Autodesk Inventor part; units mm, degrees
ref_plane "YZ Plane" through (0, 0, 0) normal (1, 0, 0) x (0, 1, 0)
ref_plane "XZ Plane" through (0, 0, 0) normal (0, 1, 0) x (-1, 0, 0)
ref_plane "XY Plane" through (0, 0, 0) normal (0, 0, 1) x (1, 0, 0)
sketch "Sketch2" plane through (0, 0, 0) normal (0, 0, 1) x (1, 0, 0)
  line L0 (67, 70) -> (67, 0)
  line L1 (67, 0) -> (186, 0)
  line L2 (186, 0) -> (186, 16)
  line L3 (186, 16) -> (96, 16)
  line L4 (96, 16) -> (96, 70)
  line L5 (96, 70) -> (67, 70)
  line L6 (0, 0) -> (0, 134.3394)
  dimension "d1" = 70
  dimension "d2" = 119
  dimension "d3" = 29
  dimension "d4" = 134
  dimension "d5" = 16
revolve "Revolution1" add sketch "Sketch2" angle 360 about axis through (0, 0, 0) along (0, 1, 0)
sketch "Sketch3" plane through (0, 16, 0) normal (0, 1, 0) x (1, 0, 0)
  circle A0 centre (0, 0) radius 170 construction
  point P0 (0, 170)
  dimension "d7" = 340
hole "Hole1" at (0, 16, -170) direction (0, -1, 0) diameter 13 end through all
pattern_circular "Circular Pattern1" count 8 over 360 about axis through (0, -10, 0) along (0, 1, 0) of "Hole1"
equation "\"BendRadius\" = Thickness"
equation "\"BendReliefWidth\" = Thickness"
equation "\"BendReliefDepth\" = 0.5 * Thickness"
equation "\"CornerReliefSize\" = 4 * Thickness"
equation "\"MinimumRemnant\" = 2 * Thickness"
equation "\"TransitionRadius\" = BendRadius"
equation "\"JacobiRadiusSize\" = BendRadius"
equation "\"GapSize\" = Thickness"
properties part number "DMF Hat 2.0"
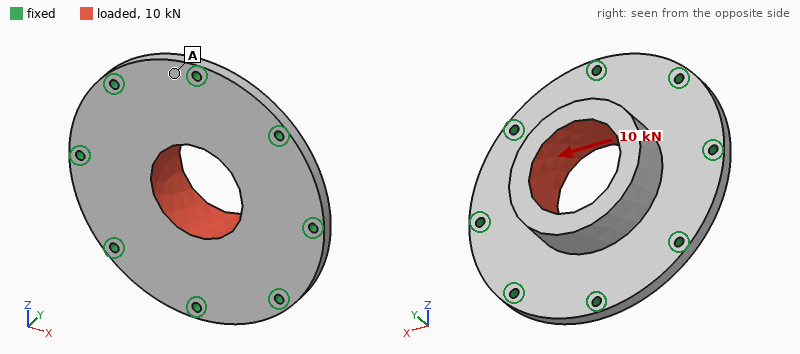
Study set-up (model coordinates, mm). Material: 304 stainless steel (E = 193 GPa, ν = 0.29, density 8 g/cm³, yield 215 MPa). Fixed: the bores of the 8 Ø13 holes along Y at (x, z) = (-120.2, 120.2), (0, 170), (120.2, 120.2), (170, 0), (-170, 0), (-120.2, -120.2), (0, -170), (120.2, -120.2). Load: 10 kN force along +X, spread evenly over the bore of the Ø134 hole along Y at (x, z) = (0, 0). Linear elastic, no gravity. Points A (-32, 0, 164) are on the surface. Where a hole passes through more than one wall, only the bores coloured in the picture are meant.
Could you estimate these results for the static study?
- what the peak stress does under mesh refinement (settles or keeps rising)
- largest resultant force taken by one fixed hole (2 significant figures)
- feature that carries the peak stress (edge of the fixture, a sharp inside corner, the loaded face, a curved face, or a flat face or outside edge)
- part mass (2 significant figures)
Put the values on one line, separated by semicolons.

keeps rising; 1.9 kN; edge of the fixture; 18 kg
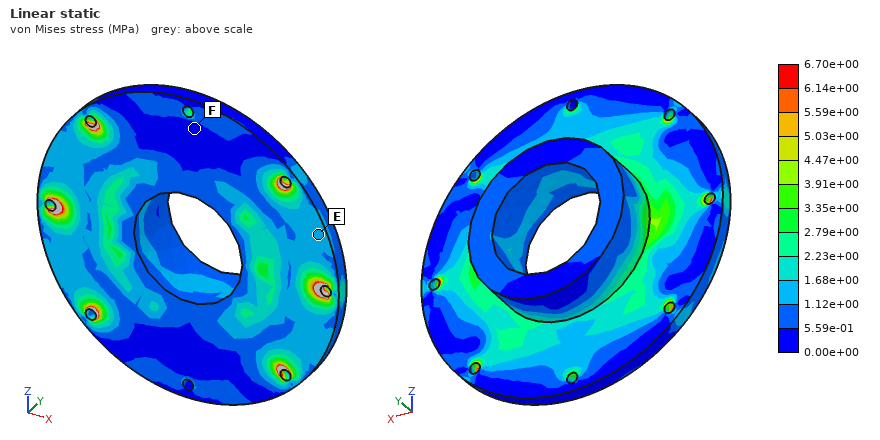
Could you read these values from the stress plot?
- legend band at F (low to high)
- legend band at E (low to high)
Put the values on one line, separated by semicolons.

0.00e+00 to 5.59e-01 MPa; 1.12e+00 to 1.68e+00 MPa
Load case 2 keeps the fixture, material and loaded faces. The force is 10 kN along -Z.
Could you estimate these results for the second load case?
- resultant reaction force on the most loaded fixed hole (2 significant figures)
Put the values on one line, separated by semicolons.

1.9 kN
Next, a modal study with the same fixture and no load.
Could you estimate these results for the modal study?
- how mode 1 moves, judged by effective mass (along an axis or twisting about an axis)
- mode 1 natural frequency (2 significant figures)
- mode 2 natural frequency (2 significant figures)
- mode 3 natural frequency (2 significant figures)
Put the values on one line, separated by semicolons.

along Y; 1300 Hz; 1900 Hz; 1900 Hz
